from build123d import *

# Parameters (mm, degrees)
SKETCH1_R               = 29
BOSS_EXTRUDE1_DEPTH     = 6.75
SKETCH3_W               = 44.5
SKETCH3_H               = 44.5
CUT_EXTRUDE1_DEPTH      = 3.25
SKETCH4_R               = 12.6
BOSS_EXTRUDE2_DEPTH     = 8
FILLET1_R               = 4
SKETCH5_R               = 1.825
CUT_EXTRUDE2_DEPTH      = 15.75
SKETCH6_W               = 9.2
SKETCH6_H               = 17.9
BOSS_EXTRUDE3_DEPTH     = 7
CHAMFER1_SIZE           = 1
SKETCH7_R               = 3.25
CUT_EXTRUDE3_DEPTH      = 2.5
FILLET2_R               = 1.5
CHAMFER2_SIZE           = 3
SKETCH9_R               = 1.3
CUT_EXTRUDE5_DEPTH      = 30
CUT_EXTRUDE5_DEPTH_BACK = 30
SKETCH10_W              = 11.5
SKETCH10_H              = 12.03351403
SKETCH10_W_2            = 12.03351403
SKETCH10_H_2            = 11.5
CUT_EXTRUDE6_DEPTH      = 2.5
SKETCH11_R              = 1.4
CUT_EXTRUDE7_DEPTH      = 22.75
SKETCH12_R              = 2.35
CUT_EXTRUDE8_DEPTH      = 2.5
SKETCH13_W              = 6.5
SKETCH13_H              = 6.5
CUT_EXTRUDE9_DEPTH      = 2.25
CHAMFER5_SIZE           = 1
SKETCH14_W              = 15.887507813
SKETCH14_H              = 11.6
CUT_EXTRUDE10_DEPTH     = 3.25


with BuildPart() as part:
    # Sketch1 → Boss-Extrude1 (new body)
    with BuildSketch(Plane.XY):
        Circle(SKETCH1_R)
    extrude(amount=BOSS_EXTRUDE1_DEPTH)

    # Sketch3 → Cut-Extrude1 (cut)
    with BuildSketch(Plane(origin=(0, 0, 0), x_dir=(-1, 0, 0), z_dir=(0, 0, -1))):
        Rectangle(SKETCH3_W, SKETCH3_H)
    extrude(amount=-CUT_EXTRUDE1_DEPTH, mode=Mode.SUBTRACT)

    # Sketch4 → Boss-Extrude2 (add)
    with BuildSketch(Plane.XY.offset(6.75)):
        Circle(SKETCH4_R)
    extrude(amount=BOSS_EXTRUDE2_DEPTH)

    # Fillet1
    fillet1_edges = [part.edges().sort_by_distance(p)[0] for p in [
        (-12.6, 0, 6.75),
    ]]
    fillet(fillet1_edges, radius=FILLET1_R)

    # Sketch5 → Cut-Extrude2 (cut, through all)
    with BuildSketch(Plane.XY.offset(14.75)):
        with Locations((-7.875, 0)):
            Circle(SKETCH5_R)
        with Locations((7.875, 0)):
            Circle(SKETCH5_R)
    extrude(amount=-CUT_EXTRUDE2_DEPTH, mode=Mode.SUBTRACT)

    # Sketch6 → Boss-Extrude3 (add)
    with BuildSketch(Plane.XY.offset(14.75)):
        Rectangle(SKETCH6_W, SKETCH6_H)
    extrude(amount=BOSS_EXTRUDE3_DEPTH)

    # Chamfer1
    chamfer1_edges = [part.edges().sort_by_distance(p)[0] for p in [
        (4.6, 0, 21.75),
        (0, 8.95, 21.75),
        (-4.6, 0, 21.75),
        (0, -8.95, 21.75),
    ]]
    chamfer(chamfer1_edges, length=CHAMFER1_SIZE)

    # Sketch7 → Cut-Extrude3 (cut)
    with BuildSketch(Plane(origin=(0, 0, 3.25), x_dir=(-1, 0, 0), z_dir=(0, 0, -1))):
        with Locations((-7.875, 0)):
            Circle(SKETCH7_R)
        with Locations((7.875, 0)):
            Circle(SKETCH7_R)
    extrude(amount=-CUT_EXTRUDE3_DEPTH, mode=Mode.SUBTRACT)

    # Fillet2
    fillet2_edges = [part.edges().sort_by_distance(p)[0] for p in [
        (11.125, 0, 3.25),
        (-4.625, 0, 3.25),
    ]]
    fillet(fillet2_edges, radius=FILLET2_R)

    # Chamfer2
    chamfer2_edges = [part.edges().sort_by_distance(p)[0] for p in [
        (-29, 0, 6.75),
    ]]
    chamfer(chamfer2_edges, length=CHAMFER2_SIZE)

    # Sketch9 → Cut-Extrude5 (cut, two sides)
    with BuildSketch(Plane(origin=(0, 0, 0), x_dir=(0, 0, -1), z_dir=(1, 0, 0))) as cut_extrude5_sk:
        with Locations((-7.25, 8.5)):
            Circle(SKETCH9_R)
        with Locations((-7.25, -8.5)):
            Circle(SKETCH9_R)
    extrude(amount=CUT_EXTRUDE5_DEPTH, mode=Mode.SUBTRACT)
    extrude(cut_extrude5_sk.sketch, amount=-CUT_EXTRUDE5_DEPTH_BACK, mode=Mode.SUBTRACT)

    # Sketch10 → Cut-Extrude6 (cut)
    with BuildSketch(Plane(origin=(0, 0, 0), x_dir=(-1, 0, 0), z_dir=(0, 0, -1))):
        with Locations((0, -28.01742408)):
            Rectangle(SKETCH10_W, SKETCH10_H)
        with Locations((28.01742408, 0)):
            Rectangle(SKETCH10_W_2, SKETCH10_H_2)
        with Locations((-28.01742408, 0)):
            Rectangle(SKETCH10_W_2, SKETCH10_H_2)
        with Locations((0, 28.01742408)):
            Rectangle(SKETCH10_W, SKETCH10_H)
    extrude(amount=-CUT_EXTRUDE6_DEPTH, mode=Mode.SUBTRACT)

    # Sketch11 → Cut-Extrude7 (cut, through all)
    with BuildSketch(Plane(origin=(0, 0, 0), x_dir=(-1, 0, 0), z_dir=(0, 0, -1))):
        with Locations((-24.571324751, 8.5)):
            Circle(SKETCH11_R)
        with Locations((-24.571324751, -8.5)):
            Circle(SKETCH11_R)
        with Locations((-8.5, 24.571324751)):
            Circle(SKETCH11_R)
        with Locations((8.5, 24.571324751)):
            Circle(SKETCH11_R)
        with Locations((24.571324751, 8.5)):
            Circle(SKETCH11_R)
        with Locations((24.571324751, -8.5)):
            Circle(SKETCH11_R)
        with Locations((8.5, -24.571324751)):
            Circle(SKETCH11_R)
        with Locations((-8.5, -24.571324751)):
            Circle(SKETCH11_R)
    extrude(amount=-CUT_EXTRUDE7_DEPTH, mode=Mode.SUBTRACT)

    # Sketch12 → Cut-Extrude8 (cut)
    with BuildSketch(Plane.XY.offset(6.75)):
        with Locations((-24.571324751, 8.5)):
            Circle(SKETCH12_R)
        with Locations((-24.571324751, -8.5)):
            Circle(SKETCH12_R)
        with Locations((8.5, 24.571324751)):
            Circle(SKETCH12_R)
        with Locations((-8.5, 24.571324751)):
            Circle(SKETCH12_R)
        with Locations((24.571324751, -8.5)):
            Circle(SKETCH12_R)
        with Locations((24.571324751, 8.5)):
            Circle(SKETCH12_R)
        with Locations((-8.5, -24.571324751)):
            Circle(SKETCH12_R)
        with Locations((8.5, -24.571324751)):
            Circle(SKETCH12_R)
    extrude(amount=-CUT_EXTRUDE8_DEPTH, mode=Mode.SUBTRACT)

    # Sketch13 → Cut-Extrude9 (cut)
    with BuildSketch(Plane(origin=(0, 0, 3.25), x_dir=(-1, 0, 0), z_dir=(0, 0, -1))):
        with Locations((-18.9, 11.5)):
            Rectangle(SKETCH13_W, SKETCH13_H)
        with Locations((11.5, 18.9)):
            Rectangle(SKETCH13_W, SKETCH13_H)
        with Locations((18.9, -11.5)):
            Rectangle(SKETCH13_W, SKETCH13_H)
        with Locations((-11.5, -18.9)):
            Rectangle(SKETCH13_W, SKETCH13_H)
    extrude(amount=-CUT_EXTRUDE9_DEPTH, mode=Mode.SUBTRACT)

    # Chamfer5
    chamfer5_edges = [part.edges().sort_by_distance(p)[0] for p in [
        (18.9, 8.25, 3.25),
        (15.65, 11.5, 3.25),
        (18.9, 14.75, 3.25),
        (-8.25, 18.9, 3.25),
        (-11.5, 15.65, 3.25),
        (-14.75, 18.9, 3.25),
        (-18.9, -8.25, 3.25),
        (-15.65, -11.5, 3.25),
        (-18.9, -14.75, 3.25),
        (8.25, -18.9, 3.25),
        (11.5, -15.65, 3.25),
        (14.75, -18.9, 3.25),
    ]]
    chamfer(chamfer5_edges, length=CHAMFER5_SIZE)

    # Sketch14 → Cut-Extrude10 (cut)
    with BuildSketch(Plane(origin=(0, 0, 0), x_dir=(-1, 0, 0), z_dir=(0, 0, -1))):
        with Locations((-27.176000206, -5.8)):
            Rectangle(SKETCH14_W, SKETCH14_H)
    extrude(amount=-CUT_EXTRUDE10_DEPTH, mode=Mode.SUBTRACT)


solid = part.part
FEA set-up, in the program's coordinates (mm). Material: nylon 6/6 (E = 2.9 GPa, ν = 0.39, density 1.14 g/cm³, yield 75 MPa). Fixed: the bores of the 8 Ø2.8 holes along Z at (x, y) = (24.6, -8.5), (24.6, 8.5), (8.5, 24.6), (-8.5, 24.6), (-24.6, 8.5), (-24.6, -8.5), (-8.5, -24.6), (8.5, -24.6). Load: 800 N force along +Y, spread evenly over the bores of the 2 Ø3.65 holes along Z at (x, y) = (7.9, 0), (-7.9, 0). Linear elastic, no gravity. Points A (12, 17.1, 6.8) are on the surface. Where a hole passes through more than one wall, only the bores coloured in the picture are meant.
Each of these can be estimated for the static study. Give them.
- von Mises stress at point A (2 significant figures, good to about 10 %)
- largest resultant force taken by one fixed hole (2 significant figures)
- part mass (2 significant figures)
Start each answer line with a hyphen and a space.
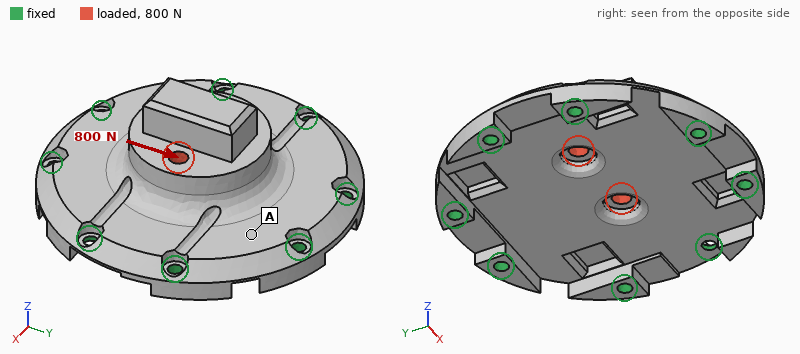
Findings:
- 2.9 MPa
- 180 N
- 16 g
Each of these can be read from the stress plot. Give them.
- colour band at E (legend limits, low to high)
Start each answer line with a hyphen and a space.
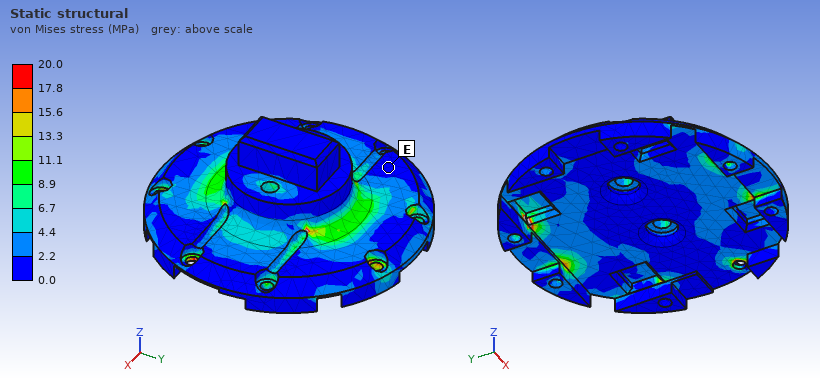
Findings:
- 0.0 to 2.2 MPa
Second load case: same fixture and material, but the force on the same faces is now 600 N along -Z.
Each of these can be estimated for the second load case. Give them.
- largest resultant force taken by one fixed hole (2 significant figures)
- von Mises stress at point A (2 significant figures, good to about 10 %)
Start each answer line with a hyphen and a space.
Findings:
- 170 N
- 4.0 MPa
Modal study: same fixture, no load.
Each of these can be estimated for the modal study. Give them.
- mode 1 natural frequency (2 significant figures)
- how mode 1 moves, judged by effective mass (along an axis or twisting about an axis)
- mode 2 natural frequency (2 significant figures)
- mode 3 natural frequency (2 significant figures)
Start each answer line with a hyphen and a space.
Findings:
- 3200 Hz
- along Z
- 4800 Hz
- 4900 Hz
